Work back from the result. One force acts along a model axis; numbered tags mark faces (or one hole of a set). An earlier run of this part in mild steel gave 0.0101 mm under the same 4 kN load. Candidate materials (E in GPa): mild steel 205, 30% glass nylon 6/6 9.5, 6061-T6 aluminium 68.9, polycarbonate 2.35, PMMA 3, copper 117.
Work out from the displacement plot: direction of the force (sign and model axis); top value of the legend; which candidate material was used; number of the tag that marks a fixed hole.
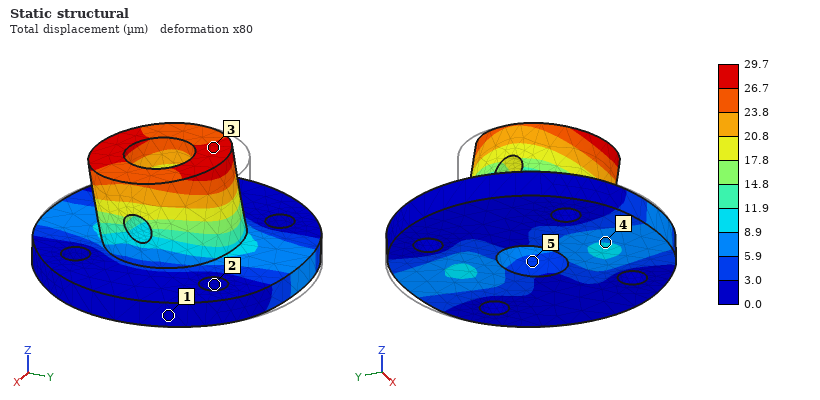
-Y
29.7 µm
6061-T6 aluminium
2
